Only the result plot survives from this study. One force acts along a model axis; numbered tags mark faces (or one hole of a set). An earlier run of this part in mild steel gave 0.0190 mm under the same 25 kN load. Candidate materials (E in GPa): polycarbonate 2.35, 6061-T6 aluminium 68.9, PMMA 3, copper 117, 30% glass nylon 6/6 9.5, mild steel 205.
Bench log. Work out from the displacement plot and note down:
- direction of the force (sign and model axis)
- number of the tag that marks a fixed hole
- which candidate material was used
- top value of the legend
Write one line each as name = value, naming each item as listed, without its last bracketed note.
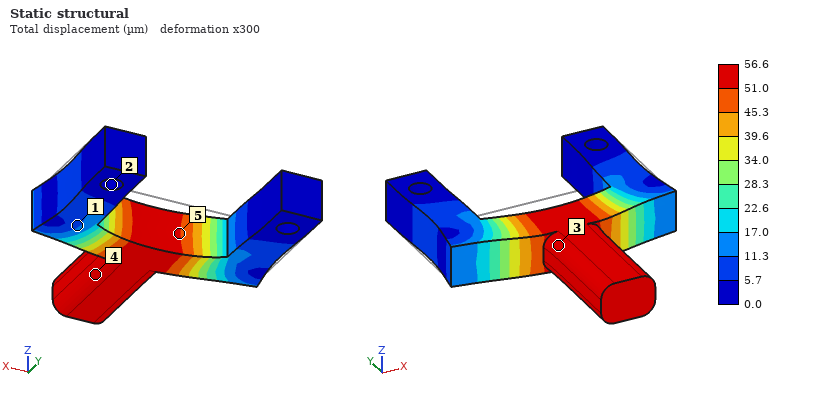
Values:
direction of the force = -Y
number of the tag that marks a fixed hole = 2
which candidate material was used = 6061-T6 aluminium
top value of the legend = 56.6 µm
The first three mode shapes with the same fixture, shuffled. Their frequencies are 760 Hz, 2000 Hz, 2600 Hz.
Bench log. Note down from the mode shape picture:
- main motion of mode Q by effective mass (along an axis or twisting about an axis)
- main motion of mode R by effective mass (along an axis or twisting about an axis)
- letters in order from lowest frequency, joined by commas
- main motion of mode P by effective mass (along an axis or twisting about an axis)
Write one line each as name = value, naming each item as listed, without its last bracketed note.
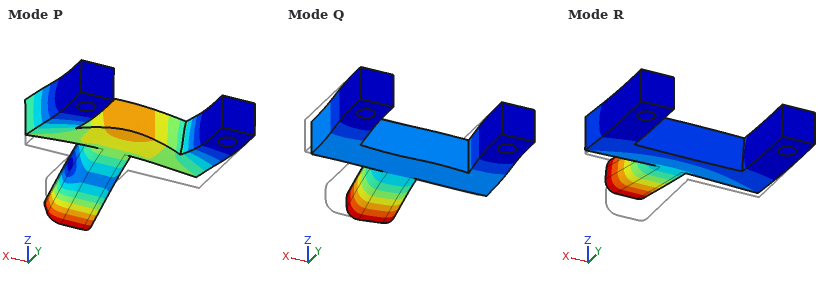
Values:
main motion of mode Q by effective mass = along X
main motion of mode R by effective mass = along Z
letters in order from lowest frequency, joined by commas = R, Q, P
main motion of mode P by effective mass = along Z
